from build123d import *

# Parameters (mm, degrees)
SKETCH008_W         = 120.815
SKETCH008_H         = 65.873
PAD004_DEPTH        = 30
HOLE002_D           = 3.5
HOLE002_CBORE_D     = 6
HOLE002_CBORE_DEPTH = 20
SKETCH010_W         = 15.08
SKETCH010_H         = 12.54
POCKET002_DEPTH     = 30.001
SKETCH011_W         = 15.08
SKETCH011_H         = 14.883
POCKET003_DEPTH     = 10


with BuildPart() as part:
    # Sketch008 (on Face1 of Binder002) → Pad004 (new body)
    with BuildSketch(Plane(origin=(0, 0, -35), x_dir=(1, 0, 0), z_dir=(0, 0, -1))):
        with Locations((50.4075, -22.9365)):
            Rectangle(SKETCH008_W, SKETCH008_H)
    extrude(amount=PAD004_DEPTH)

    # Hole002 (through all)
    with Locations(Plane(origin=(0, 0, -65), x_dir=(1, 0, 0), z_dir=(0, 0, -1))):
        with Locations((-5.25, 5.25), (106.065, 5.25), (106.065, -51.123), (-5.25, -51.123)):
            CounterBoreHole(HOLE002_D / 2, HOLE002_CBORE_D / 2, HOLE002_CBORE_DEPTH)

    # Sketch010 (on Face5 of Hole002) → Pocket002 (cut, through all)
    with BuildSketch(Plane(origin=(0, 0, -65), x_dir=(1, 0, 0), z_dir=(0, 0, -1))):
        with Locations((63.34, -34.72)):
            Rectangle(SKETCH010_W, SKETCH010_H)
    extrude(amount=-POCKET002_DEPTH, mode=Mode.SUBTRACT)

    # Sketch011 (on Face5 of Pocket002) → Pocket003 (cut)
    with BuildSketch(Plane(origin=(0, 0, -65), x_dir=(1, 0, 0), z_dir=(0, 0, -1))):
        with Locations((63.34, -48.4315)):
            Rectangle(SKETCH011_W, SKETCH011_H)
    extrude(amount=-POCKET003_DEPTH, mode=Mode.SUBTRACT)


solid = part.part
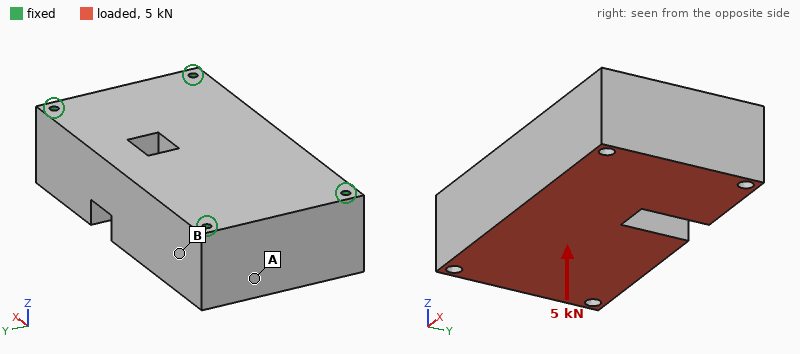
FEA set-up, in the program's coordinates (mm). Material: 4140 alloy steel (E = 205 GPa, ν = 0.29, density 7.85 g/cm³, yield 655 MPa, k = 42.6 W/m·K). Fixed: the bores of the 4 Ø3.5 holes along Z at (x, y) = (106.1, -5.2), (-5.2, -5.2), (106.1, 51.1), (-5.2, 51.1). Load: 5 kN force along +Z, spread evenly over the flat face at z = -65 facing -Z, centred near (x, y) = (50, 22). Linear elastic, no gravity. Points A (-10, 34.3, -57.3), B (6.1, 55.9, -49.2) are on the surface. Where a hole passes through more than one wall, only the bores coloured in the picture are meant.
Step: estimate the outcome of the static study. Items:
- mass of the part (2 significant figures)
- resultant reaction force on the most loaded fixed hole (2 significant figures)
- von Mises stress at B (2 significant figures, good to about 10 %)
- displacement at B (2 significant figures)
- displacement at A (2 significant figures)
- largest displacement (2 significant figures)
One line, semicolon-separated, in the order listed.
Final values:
1.8 kg; 1.6 kN; 5.2 MPa; 1.2 µm; 0.78 µm; 3.6 µm
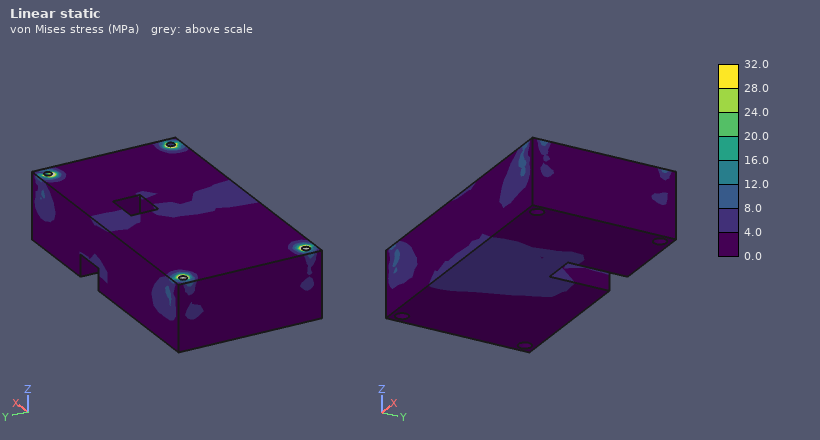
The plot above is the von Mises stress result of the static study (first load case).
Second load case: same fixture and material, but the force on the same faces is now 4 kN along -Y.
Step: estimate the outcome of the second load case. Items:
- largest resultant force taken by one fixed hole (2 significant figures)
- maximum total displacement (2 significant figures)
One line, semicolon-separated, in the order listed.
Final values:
1.5 kN; 2.1 µm
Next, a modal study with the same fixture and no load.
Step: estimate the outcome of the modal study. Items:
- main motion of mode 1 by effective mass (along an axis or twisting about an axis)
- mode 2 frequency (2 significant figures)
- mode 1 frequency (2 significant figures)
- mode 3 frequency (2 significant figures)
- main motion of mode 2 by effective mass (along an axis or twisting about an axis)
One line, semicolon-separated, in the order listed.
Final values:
along Z; 8200 Hz; 5200 Hz; 8900 Hz; along Y
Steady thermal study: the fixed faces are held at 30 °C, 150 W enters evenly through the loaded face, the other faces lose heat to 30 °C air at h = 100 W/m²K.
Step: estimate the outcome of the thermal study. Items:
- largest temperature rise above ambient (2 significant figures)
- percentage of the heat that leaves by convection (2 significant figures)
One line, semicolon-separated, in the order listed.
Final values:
44 K; 42 %
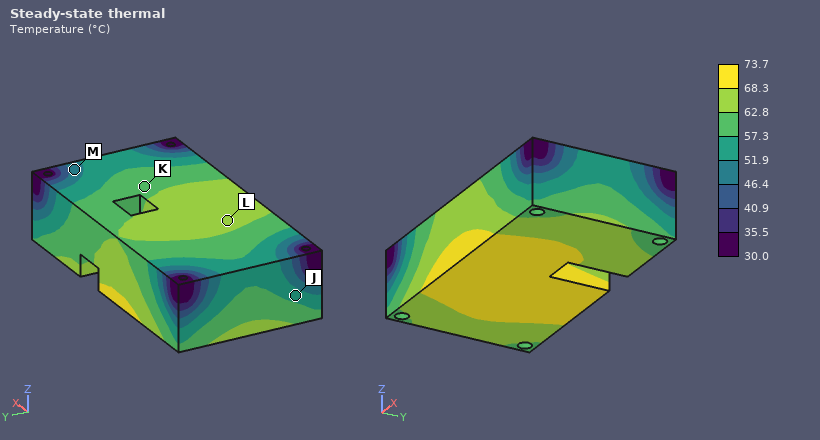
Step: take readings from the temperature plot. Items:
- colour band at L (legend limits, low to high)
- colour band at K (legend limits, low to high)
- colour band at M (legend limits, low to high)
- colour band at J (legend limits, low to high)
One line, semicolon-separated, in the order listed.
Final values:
62.8 to 68.3 °C; 57.3 to 62.8 °C; 46.4 to 51.9 °C; 51.9 to 57.3 °C
